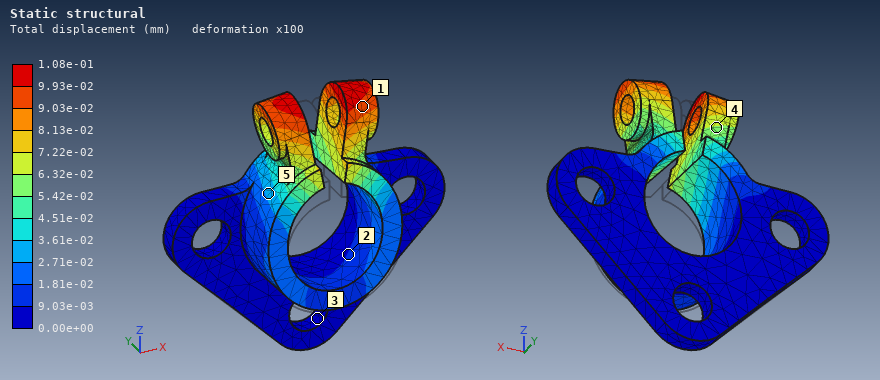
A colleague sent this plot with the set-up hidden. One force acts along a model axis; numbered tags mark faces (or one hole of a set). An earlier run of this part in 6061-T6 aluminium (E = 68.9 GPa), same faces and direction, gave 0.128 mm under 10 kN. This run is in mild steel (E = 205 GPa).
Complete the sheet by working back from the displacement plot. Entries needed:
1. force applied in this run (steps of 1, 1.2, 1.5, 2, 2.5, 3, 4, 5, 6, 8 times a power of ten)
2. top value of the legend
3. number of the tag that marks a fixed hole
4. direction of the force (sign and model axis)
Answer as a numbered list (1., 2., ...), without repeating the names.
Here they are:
1. 25 kN
2. 1.08e-01 mm
3. 3
4. +Z
